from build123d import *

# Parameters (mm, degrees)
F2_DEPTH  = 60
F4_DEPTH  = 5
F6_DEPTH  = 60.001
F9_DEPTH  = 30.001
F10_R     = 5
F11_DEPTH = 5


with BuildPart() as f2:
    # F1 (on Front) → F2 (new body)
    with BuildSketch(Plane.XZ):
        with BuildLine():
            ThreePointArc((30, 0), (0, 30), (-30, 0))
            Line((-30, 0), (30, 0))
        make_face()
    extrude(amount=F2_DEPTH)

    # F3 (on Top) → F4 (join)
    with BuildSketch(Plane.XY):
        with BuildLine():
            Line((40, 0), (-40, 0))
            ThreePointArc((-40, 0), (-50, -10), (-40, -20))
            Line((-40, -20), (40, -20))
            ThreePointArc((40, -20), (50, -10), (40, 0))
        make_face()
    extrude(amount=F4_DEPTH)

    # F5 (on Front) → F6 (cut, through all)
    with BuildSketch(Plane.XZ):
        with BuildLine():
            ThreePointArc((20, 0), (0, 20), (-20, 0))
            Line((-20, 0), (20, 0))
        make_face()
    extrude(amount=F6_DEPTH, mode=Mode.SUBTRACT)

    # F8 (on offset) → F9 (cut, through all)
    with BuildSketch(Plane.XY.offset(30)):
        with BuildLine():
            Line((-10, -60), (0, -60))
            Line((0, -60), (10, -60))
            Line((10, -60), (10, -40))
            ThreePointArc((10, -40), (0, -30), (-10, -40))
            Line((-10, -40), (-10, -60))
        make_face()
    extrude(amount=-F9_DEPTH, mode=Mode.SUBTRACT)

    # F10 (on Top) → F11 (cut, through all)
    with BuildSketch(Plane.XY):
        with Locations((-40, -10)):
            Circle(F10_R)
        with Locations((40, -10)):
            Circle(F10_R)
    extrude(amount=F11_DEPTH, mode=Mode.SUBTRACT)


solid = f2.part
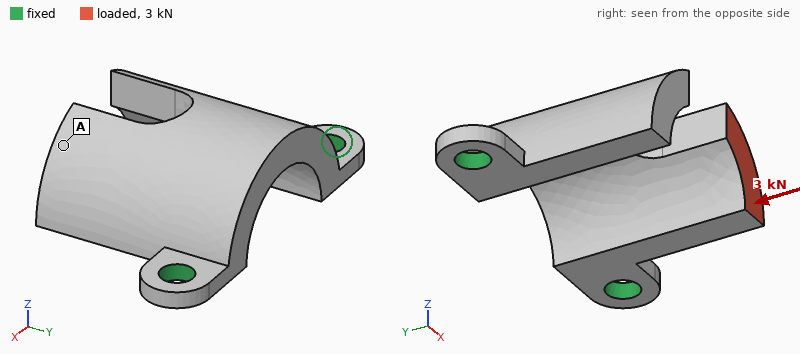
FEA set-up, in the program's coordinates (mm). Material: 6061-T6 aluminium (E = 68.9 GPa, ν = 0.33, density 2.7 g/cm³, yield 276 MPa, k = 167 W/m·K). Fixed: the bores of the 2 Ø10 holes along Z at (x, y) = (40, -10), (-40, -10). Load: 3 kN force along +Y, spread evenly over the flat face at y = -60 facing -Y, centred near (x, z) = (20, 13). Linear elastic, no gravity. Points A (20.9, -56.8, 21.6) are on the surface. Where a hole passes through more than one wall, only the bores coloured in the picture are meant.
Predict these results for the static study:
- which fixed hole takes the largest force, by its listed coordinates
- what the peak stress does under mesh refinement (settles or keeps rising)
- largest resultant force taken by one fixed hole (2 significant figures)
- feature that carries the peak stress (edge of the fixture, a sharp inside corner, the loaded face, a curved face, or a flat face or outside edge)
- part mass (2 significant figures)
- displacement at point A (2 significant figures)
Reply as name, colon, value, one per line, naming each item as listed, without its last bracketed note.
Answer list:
which fixed hole takes the largest force, by its listed coordinates: (40, -10)
what the peak stress does under mesh refinement: keeps rising
largest resultant force taken by one fixed hole: 2.4 kN
feature that carries the peak stress: edge of the fixture
part mass: 120 g
displacement at point A: 0.25 mm
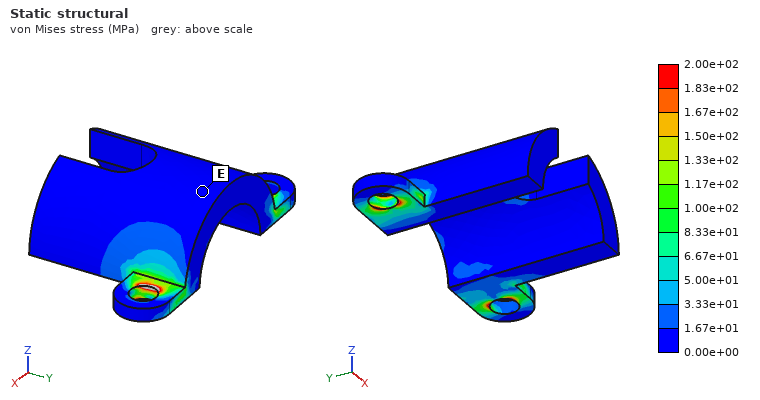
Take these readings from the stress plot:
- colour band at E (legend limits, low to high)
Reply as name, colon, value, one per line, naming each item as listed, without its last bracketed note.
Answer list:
colour band at E: 0.00e+00 to 1.67e+01 MPa
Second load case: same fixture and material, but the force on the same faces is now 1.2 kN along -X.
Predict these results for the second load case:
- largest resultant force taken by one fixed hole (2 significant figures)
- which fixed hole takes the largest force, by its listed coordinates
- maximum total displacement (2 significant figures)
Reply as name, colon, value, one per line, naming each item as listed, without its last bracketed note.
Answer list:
largest resultant force taken by one fixed hole: 1.0 kN
which fixed hole takes the largest force, by its listed coordinates: (40, -10)
maximum total displacement: 0.19 mm
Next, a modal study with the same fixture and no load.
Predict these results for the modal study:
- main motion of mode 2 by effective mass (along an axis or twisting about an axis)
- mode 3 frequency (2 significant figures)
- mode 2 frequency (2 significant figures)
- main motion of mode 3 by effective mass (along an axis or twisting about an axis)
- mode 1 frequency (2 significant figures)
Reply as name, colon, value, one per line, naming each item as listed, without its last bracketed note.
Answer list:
main motion of mode 2 by effective mass: along X
mode 3 frequency: 4700 Hz
mode 2 frequency: 3000 Hz
main motion of mode 3 by effective mass: along Y
mode 1 frequency: 1400 Hz
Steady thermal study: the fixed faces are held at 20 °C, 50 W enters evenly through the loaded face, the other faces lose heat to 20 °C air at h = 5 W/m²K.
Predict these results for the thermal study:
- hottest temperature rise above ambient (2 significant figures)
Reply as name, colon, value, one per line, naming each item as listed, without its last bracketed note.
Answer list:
hottest temperature rise above ambient: 65 K
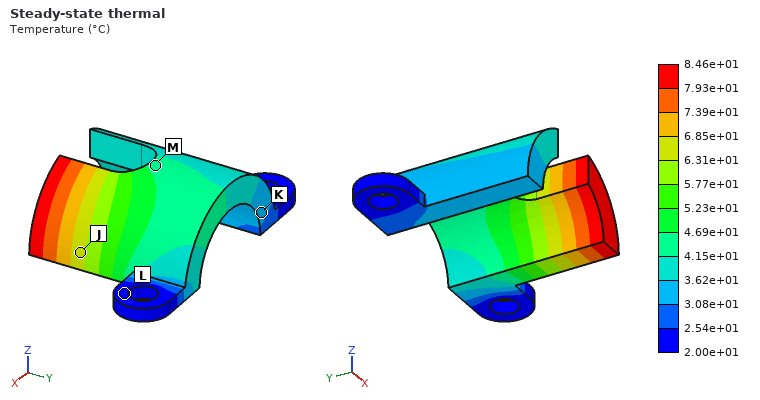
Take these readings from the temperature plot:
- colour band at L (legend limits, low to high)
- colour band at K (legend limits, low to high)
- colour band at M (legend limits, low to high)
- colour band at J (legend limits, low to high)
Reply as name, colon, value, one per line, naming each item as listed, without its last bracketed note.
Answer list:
colour band at L: 2.00e+01 to 2.54e+01 °C
colour band at K: 3.08e+01 to 3.62e+01 °C
colour band at M: 4.15e+01 to 4.69e+01 °C
colour band at J: 6.31e+01 to 6.85e+01 °C
